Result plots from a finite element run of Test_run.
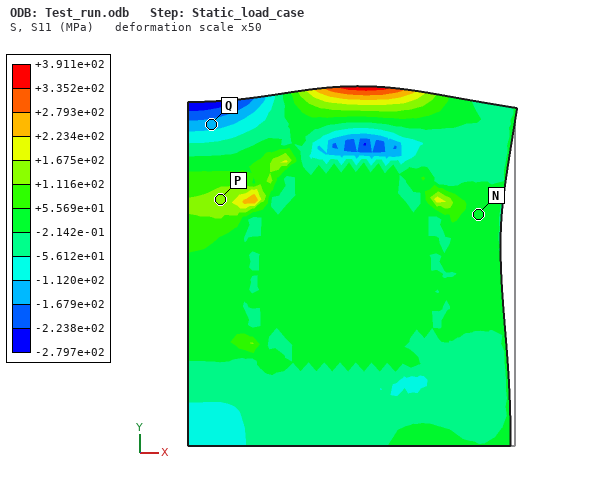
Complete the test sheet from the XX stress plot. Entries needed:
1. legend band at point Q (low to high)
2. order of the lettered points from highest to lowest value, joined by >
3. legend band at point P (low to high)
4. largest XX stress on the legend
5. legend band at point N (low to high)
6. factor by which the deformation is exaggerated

-1.679e+02 to -1.120e+02 MPa
P > N > Q
+1.116e+02 to +1.675e+02 MPa
+3.911e+02 MPa
-2.142e-01 to +5.569e+01 MPa
50
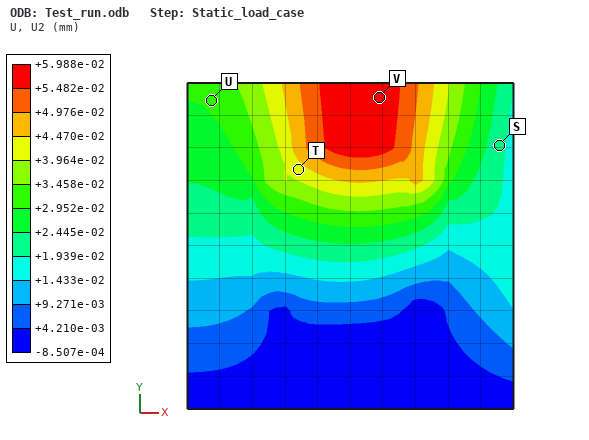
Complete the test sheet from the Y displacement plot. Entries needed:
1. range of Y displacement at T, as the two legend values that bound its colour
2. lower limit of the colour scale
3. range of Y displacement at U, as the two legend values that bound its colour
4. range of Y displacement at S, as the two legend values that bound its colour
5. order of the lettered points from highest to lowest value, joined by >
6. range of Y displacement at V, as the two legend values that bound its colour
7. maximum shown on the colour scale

+3.964e-02 to +4.470e-02 mm
-8.507e-04 mm
+2.952e-02 to +3.458e-02 mm
+1.939e-02 to +2.445e-02 mm
V > T > U > S
+5.482e-02 to +5.988e-02 mm
+5.988e-02 mm
